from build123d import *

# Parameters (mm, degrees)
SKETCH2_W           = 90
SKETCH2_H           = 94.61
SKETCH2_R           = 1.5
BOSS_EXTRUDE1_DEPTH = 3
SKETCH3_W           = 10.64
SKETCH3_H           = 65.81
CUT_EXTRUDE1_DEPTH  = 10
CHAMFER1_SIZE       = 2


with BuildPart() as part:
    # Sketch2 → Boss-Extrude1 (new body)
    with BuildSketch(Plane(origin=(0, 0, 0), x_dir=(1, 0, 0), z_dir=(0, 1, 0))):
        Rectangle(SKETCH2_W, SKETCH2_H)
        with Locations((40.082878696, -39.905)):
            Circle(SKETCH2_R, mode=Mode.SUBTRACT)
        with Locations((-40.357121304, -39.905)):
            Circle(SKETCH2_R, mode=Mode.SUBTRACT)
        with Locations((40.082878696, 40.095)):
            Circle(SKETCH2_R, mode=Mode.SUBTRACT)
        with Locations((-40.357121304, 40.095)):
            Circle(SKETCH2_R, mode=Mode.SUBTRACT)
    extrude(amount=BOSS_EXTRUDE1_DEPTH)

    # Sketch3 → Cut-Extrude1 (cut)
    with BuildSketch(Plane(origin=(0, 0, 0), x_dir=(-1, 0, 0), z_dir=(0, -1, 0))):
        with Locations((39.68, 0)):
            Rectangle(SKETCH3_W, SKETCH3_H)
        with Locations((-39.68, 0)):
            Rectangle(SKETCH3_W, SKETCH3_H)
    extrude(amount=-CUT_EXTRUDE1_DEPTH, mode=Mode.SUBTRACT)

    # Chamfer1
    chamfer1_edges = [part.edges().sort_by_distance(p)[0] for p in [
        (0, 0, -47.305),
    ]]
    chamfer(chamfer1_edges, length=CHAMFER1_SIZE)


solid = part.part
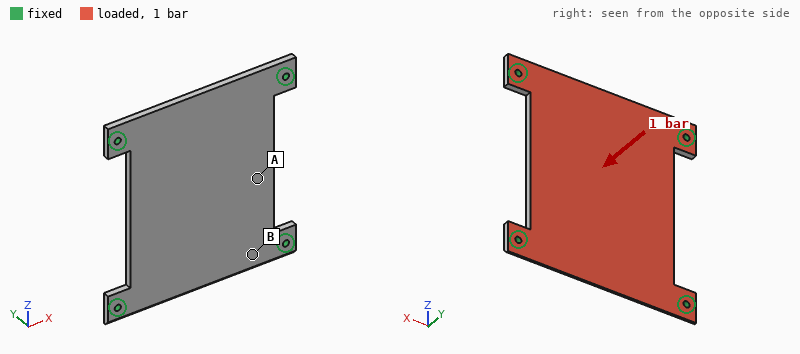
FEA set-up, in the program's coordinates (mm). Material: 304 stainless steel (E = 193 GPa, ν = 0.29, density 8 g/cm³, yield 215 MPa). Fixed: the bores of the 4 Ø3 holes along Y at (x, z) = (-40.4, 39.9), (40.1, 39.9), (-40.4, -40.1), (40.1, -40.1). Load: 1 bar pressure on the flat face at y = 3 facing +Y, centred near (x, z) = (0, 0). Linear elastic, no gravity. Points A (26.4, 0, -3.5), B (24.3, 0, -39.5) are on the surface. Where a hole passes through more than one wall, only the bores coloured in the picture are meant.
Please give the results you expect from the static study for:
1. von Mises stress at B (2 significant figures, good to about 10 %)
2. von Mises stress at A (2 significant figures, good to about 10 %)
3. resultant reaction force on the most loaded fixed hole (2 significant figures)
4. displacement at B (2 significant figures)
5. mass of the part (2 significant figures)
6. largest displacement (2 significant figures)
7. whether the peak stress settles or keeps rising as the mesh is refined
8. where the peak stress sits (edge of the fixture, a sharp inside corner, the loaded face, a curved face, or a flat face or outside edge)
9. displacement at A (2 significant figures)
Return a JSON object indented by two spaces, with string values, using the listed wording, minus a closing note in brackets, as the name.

{
  "von Mises stress at B": "12 MPa",
  "von Mises stress at A": "27 MPa",
  "resultant reaction force on the most loaded fixed hole": "180 N",
  "displacement at B": "22 µm",
  "mass of the part": "170 g",
  "largest displacement": "83 µm",
  "whether the peak stress settles or keeps rising as the mesh is refined": "keeps rising",
  "where the peak stress sits": "edge of the fixture",
  "displacement at A": "66 µm"
}
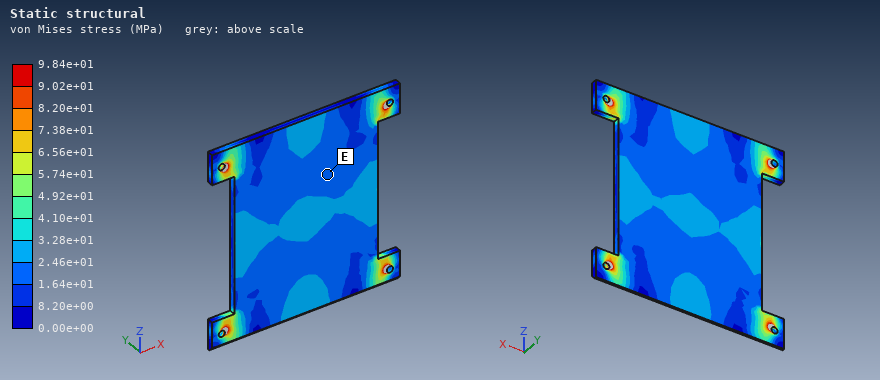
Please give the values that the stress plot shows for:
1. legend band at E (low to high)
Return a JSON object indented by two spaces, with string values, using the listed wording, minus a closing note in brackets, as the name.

{
  "legend band at E": "1.64e+01 to 2.46e+01 MPa"
}
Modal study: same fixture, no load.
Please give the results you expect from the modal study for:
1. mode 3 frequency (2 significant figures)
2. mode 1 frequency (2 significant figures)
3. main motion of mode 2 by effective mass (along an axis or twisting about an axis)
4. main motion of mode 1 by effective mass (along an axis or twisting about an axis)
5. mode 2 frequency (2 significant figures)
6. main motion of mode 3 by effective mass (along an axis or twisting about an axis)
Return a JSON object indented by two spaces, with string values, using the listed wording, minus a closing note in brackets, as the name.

{
  "mode 3 frequency": "2600 Hz",
  "mode 1 frequency": "1300 Hz",
  "main motion of mode 2 by effective mass": "twisting about X",
  "main motion of mode 1 by effective mass": "along Y",
  "mode 2 frequency": "2400 Hz",
  "main motion of mode 3 by effective mass": "twisting about Z"
}
